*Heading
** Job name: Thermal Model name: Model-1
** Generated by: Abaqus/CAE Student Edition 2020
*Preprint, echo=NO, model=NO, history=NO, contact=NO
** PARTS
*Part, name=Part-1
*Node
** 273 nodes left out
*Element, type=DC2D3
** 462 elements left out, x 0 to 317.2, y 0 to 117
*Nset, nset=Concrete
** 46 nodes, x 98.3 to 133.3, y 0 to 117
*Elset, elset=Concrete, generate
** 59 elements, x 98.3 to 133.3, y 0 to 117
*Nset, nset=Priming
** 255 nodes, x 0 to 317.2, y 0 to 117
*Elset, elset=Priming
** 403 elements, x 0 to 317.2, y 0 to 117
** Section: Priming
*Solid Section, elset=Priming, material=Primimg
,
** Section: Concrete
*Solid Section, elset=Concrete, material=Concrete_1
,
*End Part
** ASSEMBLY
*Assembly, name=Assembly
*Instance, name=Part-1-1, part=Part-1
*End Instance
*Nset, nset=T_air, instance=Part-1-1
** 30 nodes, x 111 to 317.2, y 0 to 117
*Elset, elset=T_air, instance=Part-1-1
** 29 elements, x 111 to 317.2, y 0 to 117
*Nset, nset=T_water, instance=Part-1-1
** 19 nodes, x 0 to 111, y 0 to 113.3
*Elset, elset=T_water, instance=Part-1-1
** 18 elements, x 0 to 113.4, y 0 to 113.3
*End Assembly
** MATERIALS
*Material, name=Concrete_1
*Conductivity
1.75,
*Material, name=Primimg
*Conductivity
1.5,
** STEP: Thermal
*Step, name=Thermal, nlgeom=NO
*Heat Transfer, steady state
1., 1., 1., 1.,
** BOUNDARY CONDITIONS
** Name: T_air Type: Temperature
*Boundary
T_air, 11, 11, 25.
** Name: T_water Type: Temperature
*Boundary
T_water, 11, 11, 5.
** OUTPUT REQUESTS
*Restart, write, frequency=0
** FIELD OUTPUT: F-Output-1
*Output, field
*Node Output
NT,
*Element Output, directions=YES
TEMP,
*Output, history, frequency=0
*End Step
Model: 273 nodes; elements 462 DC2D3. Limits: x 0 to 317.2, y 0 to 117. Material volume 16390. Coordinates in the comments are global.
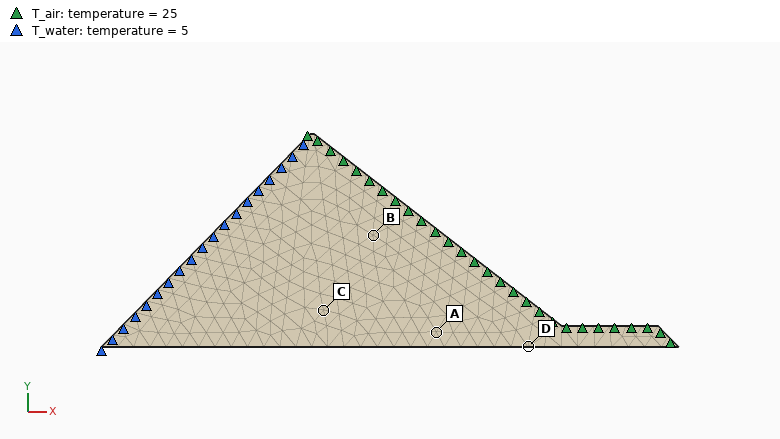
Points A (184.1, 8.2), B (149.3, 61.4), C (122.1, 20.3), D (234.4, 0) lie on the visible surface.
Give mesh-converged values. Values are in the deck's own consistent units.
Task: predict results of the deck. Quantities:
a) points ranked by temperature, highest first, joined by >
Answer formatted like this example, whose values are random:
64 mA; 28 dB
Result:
D > A > B > C
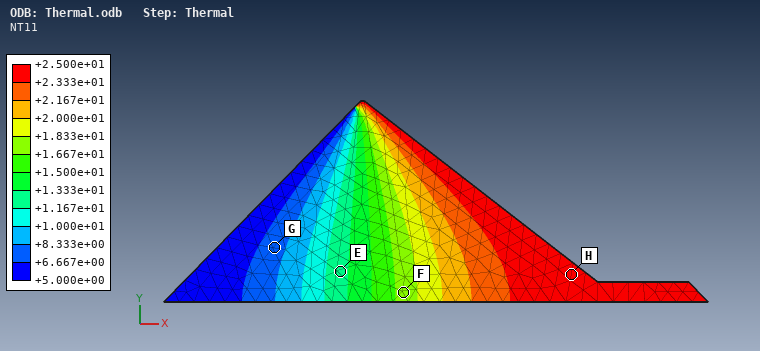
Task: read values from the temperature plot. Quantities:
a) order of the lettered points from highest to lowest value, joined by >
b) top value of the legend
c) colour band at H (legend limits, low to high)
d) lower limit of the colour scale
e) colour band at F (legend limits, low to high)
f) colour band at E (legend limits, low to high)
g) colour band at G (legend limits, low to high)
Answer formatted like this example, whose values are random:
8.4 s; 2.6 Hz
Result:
H > F > E > G; +2.500e+01; +2.333e+01 to +2.500e+01; +5.000e+00; +1.667e+01 to +1.833e+01; +1.167e+01 to +1.333e+01; +6.667e+00 to +8.333e+00
